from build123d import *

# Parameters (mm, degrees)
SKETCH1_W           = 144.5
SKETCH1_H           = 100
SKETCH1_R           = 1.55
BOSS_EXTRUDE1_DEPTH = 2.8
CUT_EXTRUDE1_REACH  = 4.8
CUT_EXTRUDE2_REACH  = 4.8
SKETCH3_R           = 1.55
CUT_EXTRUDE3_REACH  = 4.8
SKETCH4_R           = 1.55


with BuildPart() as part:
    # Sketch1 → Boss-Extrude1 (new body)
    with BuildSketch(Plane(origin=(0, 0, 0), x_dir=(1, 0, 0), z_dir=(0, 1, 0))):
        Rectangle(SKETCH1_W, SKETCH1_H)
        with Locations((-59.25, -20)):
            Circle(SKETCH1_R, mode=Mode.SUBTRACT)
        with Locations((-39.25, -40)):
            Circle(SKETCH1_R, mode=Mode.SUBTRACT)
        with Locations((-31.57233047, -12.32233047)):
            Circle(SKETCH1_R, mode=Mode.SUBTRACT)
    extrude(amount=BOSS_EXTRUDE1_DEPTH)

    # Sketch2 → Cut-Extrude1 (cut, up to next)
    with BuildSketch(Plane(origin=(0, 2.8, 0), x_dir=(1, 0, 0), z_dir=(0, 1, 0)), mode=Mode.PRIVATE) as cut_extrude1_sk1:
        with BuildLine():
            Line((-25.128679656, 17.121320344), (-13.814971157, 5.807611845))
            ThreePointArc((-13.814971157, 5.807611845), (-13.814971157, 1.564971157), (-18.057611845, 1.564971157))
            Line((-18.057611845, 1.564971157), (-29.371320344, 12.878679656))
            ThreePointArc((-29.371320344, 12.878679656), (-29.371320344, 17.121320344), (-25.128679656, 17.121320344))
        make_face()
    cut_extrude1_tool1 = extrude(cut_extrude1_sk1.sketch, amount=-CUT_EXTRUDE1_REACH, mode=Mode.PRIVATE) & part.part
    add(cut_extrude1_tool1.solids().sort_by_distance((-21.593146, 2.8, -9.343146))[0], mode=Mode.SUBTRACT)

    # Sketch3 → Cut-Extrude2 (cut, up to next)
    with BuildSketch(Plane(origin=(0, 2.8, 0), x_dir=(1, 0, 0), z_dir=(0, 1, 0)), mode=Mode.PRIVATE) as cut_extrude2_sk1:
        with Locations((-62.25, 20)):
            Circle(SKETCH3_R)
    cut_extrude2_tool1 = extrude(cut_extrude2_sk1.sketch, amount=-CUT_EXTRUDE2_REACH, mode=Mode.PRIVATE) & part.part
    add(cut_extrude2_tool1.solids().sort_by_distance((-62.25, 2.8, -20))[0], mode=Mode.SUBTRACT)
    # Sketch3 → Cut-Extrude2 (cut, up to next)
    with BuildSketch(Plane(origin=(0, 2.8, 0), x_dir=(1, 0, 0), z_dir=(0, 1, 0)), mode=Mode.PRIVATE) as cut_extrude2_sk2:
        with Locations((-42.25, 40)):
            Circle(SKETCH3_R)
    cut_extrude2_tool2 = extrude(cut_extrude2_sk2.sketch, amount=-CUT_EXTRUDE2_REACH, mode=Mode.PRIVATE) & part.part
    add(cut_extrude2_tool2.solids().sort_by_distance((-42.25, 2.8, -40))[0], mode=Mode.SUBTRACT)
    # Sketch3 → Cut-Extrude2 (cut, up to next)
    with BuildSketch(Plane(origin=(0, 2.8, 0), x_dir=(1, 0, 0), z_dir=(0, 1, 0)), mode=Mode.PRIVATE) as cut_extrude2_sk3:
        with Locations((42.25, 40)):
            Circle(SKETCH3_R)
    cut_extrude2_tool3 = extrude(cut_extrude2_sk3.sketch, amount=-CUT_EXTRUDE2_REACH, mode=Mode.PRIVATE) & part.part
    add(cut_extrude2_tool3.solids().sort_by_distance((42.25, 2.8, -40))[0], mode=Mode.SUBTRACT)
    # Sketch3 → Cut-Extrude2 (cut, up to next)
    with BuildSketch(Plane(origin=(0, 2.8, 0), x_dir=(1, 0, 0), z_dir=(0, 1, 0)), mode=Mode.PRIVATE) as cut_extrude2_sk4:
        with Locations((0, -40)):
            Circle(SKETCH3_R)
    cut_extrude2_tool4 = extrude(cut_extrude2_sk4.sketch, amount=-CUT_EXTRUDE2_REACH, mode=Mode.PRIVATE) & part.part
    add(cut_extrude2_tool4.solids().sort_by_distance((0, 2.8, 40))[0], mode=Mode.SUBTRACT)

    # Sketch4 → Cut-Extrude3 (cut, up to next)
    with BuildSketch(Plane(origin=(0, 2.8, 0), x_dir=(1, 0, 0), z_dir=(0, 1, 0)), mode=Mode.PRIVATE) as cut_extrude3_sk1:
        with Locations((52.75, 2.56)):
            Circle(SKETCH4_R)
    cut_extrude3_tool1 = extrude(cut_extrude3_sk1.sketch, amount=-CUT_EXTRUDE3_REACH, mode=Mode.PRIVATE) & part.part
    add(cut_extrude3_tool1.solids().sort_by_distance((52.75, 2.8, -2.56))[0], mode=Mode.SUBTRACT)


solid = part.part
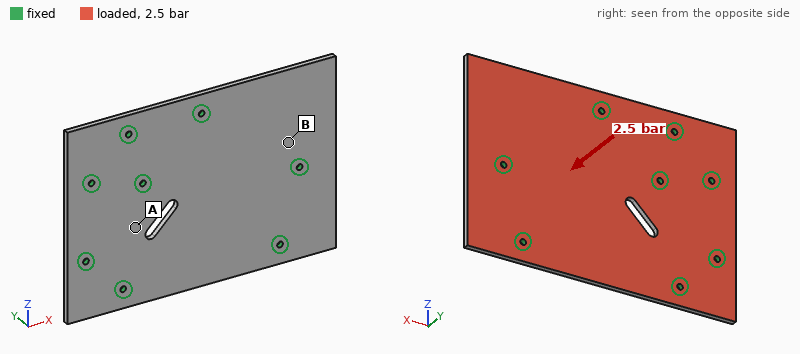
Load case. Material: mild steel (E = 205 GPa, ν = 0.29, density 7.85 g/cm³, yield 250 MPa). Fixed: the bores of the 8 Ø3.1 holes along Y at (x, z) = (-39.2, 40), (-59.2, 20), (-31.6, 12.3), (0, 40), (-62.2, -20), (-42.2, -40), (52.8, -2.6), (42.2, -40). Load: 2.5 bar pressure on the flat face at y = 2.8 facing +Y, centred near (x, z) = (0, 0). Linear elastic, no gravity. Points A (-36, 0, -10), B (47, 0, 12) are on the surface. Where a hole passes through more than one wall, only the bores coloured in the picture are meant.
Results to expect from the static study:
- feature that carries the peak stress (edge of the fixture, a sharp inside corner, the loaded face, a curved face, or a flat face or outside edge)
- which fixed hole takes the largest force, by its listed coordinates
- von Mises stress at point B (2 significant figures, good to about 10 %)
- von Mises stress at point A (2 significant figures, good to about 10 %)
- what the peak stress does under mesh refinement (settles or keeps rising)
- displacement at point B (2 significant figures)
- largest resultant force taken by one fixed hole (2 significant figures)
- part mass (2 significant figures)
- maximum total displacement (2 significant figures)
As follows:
edge of the fixture
(52.8, -2.6)
78 MPa
36 MPa
keeps rising
0.058 mm
880 N
310 g
0.37 mm
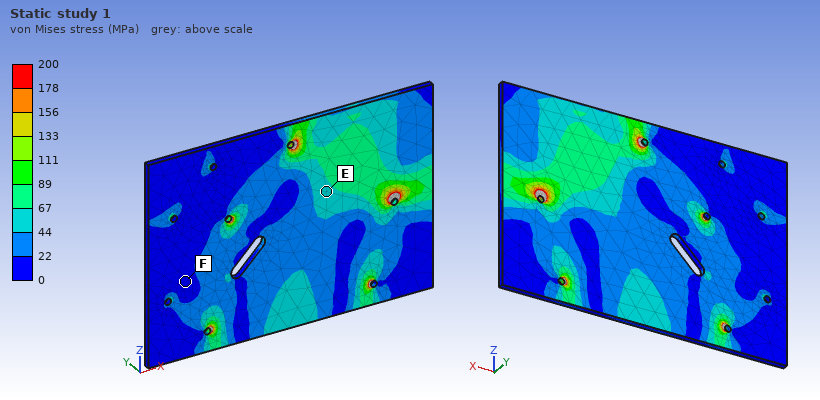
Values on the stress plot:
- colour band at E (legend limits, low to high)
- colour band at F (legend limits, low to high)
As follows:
44 to 67 MPa
0 to 22 MPa
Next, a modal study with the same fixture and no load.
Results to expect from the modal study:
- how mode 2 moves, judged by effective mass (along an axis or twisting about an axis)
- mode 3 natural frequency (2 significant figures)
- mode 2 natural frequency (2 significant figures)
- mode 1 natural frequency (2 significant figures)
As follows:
along Y
2900 Hz
2000 Hz
1200 Hz
